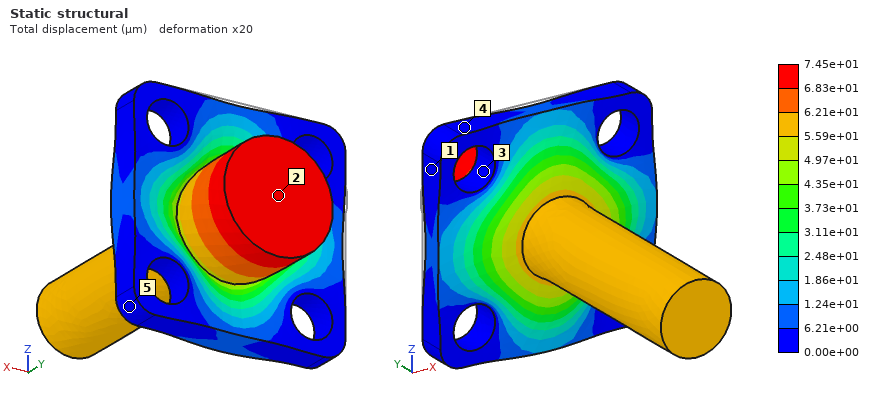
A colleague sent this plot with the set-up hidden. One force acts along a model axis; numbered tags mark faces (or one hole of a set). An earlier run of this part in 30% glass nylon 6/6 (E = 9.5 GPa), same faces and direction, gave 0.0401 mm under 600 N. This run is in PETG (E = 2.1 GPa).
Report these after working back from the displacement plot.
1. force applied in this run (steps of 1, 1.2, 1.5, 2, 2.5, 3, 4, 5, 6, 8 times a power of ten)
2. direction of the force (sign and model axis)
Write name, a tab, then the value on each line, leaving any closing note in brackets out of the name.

force applied in this run	250 N
direction of the force	-Y
